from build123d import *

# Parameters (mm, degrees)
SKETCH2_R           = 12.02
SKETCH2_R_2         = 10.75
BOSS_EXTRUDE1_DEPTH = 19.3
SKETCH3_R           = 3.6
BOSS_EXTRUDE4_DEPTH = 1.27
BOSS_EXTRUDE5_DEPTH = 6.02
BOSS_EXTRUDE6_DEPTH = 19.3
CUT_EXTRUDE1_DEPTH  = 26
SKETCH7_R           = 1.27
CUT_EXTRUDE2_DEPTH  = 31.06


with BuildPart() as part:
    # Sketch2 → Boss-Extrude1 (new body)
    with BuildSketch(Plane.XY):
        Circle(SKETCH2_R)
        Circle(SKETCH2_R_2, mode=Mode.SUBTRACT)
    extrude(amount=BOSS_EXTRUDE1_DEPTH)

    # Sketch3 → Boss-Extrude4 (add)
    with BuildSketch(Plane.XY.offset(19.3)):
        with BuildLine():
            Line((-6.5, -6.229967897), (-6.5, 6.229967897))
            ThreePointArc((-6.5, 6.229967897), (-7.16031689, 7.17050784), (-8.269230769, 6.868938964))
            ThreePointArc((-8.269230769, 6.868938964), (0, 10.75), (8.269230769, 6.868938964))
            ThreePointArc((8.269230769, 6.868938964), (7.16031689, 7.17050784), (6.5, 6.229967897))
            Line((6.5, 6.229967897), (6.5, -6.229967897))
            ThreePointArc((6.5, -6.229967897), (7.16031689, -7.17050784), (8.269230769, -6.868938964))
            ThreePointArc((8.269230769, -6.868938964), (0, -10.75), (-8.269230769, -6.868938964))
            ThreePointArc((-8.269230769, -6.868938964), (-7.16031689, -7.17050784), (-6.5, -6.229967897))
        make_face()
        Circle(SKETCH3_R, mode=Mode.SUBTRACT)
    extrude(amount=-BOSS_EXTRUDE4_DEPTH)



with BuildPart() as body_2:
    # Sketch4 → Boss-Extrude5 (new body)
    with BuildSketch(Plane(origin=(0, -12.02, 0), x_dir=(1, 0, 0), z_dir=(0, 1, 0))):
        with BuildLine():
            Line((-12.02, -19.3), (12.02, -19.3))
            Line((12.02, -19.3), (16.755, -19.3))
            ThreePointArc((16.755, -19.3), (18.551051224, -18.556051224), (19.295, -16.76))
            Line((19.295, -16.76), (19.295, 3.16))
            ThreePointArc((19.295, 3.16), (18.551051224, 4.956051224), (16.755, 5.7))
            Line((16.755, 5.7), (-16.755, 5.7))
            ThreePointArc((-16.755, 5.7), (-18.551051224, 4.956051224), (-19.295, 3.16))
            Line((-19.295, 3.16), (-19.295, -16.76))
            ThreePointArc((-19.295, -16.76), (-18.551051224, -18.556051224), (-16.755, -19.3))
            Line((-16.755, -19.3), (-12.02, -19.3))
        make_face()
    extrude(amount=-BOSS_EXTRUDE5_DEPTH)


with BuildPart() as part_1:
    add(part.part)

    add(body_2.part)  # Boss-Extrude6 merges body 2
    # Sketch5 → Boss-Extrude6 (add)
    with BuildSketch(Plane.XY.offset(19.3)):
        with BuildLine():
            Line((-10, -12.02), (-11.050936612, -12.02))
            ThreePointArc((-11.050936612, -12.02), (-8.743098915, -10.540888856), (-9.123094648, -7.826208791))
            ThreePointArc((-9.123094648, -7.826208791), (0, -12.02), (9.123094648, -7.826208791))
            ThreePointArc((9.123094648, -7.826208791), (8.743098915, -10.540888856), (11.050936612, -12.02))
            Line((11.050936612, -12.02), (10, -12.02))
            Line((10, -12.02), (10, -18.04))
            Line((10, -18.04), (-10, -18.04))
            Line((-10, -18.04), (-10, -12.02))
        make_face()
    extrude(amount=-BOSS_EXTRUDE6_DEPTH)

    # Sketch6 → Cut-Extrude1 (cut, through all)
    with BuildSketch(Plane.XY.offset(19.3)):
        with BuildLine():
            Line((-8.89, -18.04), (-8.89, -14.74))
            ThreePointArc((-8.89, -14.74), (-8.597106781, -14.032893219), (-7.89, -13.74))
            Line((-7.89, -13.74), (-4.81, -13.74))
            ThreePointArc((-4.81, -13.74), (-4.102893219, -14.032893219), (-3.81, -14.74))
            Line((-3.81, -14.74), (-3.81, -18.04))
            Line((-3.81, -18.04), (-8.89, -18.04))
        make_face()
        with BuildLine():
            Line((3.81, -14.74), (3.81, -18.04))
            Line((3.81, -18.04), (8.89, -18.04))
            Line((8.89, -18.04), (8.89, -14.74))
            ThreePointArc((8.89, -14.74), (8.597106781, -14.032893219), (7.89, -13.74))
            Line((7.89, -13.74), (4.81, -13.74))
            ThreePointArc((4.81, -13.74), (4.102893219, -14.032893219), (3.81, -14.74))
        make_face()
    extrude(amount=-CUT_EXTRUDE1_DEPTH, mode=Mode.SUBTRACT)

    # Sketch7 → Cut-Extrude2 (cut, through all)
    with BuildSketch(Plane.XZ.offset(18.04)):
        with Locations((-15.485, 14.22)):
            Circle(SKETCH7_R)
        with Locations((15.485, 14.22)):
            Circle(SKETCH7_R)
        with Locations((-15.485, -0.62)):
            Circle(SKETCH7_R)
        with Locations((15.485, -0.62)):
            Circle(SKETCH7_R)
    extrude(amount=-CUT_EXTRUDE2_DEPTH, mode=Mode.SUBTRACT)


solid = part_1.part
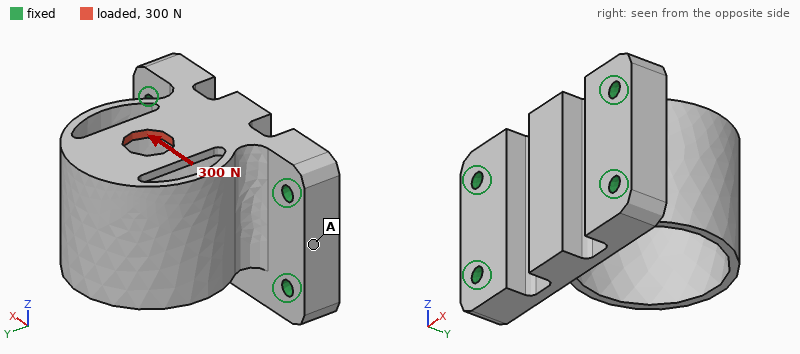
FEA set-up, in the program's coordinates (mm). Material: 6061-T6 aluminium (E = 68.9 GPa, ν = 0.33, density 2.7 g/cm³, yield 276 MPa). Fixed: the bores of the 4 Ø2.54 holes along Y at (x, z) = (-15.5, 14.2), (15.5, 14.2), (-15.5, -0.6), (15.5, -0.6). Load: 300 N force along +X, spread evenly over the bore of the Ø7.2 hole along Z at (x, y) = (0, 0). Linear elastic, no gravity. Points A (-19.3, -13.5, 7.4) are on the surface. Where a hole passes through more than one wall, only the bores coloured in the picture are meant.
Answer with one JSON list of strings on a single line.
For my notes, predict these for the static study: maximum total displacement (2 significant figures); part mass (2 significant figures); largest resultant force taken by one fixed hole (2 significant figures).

["38 µm", "19 g", "220 N"]
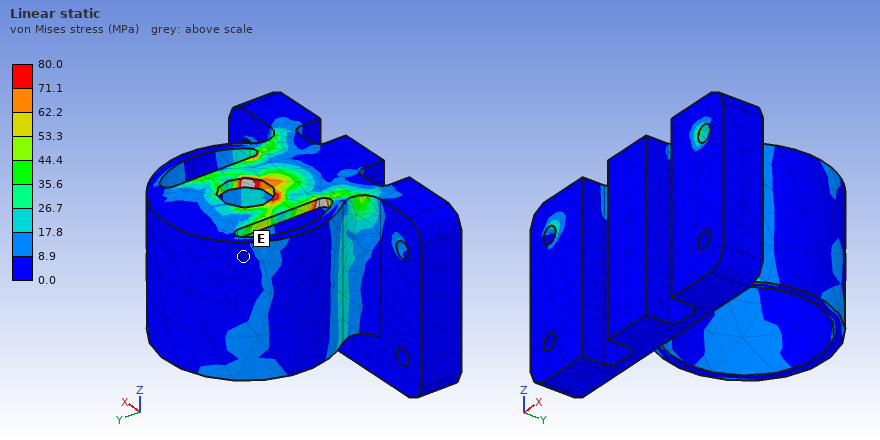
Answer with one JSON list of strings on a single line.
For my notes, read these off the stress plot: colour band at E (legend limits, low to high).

["0.0 to 8.9 MPa"]
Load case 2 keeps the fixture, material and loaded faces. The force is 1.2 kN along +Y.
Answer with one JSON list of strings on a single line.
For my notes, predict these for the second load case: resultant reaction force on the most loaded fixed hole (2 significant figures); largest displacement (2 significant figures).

["890 N", "53 µm"]
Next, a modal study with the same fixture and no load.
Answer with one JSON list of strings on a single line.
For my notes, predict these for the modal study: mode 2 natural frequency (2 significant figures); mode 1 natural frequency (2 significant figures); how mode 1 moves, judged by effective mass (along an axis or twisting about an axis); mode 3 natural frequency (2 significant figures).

["6700 Hz", "5500 Hz", "along X", "12 kHz"]
